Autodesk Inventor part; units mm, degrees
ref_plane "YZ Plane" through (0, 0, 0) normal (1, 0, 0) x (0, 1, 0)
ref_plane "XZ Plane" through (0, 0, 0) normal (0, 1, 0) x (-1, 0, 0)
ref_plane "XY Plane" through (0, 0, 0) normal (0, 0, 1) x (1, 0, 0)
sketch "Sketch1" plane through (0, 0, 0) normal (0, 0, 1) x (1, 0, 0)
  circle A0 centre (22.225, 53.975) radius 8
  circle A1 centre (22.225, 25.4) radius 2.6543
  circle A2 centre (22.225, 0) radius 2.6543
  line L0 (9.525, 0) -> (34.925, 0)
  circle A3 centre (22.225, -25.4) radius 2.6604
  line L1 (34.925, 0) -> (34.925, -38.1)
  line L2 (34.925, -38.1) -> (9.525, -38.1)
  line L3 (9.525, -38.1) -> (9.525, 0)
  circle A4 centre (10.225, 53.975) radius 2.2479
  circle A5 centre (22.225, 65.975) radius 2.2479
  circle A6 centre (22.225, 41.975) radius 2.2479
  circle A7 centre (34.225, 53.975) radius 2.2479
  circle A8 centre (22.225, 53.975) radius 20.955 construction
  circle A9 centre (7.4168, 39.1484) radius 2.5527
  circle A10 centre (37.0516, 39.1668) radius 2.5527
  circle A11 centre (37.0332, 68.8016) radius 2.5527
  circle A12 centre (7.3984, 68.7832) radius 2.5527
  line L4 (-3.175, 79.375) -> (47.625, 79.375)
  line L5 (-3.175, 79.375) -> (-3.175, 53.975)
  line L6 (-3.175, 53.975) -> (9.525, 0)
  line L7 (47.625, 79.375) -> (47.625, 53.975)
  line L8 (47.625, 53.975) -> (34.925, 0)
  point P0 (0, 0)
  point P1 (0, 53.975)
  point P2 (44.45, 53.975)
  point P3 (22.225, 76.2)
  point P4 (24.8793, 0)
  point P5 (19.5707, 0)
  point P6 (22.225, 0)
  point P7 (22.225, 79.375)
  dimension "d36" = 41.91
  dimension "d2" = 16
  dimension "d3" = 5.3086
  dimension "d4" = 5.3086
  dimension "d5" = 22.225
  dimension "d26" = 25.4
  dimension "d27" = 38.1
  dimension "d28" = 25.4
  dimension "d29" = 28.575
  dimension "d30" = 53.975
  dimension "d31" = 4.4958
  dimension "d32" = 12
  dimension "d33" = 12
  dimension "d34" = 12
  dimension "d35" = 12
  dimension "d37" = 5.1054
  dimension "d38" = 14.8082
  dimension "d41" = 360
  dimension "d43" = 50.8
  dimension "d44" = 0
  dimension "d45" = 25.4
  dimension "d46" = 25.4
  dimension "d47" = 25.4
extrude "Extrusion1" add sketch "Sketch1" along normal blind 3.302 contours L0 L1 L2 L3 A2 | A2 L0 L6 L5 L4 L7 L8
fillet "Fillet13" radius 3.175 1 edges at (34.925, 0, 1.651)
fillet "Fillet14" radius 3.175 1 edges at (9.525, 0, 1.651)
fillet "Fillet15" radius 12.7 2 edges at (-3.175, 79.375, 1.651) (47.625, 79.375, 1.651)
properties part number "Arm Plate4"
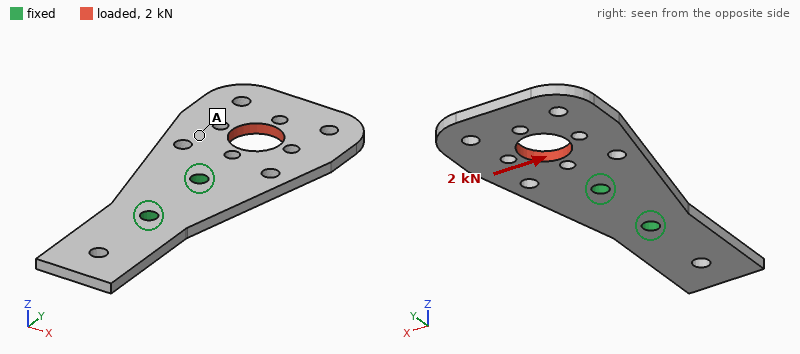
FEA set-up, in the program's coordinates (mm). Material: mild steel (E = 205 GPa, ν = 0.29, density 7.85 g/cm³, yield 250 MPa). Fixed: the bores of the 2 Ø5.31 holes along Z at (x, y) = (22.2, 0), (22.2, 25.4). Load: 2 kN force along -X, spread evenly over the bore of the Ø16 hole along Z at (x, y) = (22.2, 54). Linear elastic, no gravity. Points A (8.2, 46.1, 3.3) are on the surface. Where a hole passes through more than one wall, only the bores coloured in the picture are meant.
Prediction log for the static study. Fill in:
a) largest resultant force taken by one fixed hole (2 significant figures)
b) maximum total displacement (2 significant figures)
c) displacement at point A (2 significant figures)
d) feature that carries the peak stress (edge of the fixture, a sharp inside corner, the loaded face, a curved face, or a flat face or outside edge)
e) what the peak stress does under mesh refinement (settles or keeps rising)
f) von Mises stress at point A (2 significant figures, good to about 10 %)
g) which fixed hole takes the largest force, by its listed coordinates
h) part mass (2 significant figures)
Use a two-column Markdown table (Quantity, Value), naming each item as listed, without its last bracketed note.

| Quantity | Value |
|---|---|
| largest resultant force taken by one fixed hole | 3.7 kN |
| maximum total displacement | 52 µm |
| displacement at point A | 22 µm |
| feature that carries the peak stress | edge of the fixture |
| what the peak stress does under mesh refinement | keeps rising |
| von Mises stress at point A | 30 MPa |
| which fixed hole takes the largest force, by its listed coordinates | (22.2, 25.4) |
| part mass | 99 g |
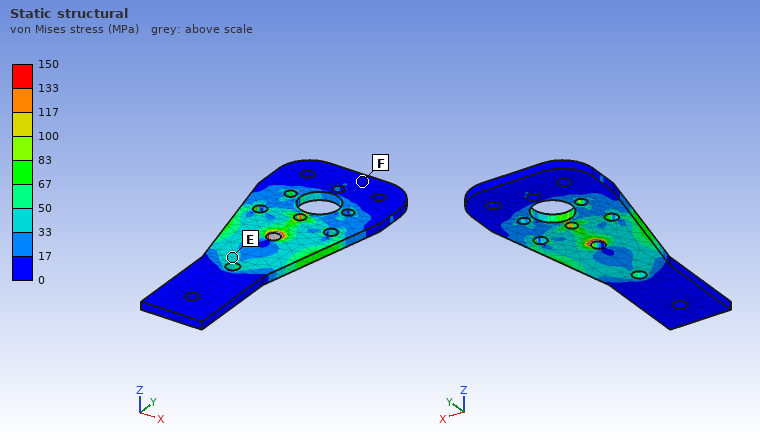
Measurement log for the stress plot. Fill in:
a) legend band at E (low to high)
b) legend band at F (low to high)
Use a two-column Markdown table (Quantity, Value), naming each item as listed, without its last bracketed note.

| Quantity | Value |
|---|---|
| legend band at E | 33 to 50 MPa |
| legend band at F | 0 to 17 MPa |
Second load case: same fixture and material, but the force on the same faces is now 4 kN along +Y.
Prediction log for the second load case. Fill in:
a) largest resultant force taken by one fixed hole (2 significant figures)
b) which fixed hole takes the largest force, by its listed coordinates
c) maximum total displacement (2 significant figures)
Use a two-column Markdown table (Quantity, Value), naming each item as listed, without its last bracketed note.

| Quantity | Value |
|---|---|
| largest resultant force taken by one fixed hole | 3.0 kN |
| which fixed hole takes the largest force, by its listed coordinates | (22.2, 25.4) |
| maximum total displacement | 12 µm |
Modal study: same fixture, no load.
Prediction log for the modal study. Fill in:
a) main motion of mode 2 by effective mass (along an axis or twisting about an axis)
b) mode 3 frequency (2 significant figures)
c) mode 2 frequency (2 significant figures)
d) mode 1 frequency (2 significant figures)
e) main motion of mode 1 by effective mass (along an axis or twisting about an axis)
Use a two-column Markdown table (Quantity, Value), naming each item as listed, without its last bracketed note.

| Quantity | Value |
|---|---|
| main motion of mode 2 by effective mass | twisting about Y |
| mode 3 frequency | 2000 Hz |
| mode 2 frequency | 1700 Hz |
| mode 1 frequency | 850 Hz |
| main motion of mode 1 by effective mass | along Z |
